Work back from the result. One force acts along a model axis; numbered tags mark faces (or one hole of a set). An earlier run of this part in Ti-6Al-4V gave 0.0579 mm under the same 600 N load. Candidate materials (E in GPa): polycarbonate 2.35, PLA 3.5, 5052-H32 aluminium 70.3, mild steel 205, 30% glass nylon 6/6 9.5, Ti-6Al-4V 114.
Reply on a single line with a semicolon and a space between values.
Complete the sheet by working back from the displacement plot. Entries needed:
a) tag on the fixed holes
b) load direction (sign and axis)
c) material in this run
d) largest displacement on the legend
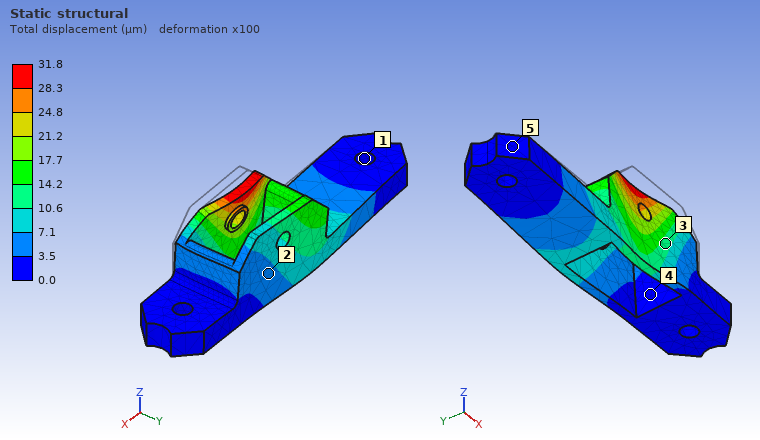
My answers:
1; +Y; mild steel; 31.8 µm
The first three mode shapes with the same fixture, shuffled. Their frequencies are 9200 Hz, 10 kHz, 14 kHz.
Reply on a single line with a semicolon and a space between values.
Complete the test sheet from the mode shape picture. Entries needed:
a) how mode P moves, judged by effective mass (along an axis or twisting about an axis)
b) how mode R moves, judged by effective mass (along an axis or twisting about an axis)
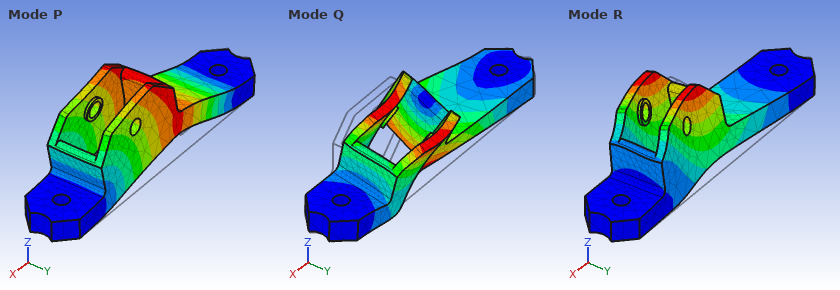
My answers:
along Z; along Y
